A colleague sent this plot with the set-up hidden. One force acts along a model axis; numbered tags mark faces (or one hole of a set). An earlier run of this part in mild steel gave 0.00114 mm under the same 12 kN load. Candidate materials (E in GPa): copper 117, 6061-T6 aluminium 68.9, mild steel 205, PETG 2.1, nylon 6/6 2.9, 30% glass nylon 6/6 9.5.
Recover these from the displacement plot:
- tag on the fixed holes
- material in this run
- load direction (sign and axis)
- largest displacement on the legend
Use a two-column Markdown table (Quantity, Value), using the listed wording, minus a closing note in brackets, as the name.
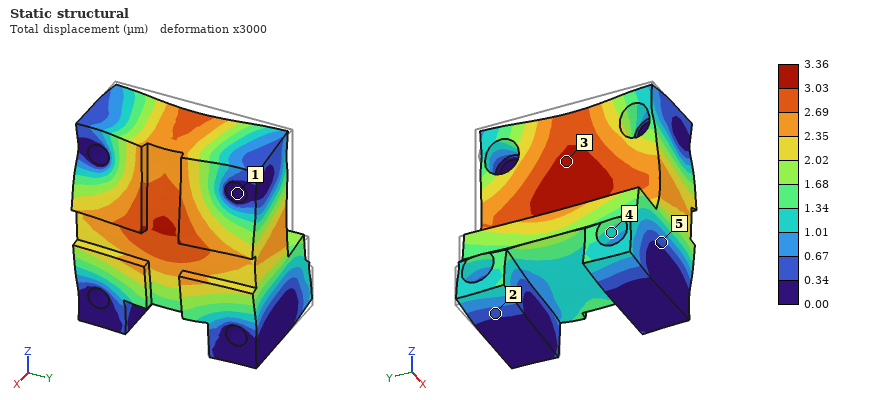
| Quantity | Value |
|---|---|
| tag on the fixed holes | 1 |
| material in this run | 6061-T6 aluminium |
| load direction | +X |
| largest displacement on the legend | 3.36 µm |
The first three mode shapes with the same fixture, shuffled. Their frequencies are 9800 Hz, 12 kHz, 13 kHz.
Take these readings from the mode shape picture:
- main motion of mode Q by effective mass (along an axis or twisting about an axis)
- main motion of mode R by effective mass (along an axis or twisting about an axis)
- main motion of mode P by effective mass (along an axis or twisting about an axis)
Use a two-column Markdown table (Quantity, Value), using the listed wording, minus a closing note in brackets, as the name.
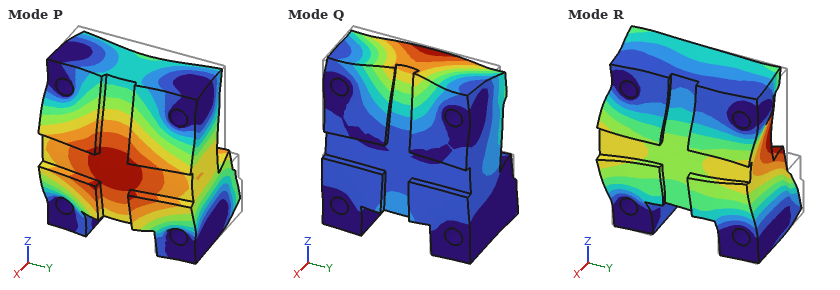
| Quantity | Value |
|---|---|
| main motion of mode Q by effective mass | along Z |
| main motion of mode R by effective mass | along Y |
| main motion of mode P by effective mass | along X |
